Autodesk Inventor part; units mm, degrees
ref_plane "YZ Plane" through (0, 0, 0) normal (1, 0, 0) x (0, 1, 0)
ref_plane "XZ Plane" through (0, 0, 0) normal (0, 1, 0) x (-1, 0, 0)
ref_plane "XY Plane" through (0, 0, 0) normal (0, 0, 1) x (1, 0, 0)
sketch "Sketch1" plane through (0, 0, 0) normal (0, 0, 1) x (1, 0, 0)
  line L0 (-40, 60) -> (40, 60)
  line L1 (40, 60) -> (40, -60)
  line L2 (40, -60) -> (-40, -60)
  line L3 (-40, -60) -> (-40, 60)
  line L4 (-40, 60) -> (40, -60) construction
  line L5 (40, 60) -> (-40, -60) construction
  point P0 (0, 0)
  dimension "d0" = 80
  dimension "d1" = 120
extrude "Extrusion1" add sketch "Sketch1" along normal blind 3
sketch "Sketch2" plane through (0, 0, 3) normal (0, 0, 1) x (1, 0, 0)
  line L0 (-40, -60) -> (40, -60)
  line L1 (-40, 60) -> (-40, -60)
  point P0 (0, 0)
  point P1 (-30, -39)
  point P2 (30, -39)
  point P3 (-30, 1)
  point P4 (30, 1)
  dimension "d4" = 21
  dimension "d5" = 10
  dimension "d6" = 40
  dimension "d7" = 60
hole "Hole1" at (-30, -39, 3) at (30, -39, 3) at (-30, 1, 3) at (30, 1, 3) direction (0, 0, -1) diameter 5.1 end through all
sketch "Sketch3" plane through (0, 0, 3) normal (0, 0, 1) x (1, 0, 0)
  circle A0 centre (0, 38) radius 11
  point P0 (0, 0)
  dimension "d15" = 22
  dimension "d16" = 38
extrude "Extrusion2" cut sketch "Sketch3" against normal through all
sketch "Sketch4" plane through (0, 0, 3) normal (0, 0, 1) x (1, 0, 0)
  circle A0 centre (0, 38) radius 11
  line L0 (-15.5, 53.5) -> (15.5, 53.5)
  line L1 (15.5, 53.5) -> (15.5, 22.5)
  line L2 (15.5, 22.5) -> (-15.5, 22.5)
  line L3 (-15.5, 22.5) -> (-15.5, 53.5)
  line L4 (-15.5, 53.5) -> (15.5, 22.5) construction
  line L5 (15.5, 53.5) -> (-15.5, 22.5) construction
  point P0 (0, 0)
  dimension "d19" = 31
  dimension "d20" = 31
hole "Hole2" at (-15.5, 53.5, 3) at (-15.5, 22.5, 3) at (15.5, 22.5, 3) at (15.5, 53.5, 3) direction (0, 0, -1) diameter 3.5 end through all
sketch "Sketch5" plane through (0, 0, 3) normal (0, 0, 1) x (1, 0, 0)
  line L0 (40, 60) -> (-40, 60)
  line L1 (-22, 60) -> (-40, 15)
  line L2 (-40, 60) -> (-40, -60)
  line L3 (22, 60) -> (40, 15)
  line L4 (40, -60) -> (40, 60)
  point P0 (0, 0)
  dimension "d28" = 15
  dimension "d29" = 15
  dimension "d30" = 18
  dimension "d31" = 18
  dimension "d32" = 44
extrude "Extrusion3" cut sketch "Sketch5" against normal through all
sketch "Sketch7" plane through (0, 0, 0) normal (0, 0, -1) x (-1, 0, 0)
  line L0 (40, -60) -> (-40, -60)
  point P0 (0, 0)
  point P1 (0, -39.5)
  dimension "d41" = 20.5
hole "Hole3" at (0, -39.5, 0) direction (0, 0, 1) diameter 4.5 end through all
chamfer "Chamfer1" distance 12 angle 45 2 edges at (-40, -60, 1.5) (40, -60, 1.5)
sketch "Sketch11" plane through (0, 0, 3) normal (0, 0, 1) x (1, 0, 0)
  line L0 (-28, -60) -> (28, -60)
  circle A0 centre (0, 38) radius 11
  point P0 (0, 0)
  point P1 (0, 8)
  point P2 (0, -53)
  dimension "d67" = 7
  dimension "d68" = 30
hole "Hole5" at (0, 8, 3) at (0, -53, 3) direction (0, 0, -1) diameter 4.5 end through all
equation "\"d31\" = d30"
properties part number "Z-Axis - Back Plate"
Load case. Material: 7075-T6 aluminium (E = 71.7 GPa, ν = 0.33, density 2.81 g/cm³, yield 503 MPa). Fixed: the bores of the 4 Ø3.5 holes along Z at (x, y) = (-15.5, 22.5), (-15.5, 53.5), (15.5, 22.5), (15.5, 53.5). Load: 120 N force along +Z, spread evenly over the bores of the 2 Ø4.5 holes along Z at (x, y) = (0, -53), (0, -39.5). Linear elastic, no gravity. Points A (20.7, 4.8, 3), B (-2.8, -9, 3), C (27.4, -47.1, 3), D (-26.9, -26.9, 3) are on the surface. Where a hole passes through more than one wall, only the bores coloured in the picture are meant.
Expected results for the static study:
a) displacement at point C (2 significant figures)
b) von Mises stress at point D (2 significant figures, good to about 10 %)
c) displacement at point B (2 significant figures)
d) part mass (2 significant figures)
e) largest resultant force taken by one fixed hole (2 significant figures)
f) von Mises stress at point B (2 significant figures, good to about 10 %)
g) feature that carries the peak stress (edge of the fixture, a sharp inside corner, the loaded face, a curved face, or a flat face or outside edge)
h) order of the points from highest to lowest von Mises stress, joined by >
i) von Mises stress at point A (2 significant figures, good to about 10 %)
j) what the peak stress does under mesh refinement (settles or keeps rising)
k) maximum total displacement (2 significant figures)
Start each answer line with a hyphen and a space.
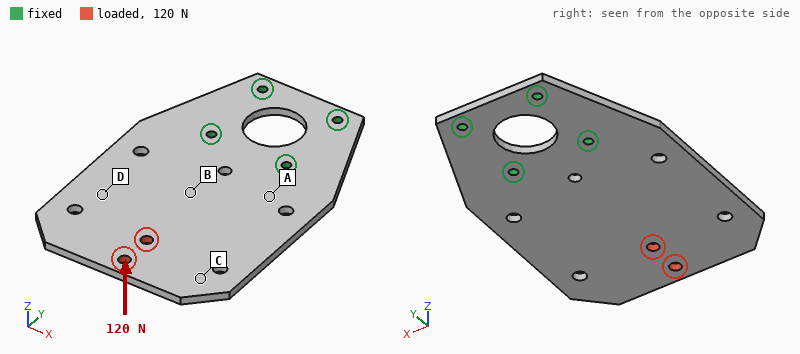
- 1.1 mm
- 20 MPa
- 0.33 mm
- 68 g
- 100 N
- 36 MPa
- edge of the fixture
- A > B > D > C
- 52 MPa
- keeps rising
- 1.5 mm
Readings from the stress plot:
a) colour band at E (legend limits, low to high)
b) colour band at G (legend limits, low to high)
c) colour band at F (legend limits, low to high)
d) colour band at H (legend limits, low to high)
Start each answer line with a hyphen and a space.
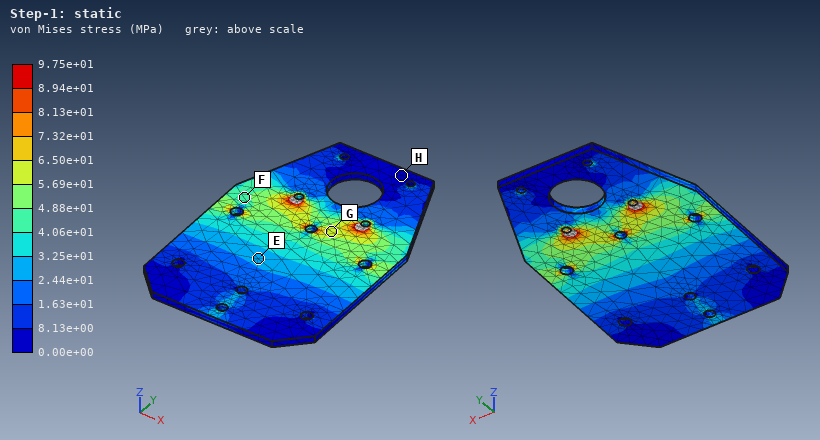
- 2.44e+01 to 3.25e+01 MPa
- 5.69e+01 to 6.50e+01 MPa
- 4.06e+01 to 4.88e+01 MPa
- 0.00e+00 to 8.13e+00 MPa
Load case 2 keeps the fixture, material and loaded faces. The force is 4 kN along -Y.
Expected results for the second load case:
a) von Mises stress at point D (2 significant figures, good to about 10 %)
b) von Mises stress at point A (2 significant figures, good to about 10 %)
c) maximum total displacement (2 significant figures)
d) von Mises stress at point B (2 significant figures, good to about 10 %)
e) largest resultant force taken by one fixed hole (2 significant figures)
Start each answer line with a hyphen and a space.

- 12 MPa
- 22 MPa
- 36 µm
- 26 MPa
- 1.7 kN
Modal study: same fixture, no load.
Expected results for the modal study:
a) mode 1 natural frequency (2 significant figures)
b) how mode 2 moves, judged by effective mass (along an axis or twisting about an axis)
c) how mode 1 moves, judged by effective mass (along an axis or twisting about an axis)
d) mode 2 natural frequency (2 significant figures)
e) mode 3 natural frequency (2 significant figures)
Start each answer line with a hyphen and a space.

- 360 Hz
- twisting about Y
- along Z
- 870 Hz
- 2000 Hz
